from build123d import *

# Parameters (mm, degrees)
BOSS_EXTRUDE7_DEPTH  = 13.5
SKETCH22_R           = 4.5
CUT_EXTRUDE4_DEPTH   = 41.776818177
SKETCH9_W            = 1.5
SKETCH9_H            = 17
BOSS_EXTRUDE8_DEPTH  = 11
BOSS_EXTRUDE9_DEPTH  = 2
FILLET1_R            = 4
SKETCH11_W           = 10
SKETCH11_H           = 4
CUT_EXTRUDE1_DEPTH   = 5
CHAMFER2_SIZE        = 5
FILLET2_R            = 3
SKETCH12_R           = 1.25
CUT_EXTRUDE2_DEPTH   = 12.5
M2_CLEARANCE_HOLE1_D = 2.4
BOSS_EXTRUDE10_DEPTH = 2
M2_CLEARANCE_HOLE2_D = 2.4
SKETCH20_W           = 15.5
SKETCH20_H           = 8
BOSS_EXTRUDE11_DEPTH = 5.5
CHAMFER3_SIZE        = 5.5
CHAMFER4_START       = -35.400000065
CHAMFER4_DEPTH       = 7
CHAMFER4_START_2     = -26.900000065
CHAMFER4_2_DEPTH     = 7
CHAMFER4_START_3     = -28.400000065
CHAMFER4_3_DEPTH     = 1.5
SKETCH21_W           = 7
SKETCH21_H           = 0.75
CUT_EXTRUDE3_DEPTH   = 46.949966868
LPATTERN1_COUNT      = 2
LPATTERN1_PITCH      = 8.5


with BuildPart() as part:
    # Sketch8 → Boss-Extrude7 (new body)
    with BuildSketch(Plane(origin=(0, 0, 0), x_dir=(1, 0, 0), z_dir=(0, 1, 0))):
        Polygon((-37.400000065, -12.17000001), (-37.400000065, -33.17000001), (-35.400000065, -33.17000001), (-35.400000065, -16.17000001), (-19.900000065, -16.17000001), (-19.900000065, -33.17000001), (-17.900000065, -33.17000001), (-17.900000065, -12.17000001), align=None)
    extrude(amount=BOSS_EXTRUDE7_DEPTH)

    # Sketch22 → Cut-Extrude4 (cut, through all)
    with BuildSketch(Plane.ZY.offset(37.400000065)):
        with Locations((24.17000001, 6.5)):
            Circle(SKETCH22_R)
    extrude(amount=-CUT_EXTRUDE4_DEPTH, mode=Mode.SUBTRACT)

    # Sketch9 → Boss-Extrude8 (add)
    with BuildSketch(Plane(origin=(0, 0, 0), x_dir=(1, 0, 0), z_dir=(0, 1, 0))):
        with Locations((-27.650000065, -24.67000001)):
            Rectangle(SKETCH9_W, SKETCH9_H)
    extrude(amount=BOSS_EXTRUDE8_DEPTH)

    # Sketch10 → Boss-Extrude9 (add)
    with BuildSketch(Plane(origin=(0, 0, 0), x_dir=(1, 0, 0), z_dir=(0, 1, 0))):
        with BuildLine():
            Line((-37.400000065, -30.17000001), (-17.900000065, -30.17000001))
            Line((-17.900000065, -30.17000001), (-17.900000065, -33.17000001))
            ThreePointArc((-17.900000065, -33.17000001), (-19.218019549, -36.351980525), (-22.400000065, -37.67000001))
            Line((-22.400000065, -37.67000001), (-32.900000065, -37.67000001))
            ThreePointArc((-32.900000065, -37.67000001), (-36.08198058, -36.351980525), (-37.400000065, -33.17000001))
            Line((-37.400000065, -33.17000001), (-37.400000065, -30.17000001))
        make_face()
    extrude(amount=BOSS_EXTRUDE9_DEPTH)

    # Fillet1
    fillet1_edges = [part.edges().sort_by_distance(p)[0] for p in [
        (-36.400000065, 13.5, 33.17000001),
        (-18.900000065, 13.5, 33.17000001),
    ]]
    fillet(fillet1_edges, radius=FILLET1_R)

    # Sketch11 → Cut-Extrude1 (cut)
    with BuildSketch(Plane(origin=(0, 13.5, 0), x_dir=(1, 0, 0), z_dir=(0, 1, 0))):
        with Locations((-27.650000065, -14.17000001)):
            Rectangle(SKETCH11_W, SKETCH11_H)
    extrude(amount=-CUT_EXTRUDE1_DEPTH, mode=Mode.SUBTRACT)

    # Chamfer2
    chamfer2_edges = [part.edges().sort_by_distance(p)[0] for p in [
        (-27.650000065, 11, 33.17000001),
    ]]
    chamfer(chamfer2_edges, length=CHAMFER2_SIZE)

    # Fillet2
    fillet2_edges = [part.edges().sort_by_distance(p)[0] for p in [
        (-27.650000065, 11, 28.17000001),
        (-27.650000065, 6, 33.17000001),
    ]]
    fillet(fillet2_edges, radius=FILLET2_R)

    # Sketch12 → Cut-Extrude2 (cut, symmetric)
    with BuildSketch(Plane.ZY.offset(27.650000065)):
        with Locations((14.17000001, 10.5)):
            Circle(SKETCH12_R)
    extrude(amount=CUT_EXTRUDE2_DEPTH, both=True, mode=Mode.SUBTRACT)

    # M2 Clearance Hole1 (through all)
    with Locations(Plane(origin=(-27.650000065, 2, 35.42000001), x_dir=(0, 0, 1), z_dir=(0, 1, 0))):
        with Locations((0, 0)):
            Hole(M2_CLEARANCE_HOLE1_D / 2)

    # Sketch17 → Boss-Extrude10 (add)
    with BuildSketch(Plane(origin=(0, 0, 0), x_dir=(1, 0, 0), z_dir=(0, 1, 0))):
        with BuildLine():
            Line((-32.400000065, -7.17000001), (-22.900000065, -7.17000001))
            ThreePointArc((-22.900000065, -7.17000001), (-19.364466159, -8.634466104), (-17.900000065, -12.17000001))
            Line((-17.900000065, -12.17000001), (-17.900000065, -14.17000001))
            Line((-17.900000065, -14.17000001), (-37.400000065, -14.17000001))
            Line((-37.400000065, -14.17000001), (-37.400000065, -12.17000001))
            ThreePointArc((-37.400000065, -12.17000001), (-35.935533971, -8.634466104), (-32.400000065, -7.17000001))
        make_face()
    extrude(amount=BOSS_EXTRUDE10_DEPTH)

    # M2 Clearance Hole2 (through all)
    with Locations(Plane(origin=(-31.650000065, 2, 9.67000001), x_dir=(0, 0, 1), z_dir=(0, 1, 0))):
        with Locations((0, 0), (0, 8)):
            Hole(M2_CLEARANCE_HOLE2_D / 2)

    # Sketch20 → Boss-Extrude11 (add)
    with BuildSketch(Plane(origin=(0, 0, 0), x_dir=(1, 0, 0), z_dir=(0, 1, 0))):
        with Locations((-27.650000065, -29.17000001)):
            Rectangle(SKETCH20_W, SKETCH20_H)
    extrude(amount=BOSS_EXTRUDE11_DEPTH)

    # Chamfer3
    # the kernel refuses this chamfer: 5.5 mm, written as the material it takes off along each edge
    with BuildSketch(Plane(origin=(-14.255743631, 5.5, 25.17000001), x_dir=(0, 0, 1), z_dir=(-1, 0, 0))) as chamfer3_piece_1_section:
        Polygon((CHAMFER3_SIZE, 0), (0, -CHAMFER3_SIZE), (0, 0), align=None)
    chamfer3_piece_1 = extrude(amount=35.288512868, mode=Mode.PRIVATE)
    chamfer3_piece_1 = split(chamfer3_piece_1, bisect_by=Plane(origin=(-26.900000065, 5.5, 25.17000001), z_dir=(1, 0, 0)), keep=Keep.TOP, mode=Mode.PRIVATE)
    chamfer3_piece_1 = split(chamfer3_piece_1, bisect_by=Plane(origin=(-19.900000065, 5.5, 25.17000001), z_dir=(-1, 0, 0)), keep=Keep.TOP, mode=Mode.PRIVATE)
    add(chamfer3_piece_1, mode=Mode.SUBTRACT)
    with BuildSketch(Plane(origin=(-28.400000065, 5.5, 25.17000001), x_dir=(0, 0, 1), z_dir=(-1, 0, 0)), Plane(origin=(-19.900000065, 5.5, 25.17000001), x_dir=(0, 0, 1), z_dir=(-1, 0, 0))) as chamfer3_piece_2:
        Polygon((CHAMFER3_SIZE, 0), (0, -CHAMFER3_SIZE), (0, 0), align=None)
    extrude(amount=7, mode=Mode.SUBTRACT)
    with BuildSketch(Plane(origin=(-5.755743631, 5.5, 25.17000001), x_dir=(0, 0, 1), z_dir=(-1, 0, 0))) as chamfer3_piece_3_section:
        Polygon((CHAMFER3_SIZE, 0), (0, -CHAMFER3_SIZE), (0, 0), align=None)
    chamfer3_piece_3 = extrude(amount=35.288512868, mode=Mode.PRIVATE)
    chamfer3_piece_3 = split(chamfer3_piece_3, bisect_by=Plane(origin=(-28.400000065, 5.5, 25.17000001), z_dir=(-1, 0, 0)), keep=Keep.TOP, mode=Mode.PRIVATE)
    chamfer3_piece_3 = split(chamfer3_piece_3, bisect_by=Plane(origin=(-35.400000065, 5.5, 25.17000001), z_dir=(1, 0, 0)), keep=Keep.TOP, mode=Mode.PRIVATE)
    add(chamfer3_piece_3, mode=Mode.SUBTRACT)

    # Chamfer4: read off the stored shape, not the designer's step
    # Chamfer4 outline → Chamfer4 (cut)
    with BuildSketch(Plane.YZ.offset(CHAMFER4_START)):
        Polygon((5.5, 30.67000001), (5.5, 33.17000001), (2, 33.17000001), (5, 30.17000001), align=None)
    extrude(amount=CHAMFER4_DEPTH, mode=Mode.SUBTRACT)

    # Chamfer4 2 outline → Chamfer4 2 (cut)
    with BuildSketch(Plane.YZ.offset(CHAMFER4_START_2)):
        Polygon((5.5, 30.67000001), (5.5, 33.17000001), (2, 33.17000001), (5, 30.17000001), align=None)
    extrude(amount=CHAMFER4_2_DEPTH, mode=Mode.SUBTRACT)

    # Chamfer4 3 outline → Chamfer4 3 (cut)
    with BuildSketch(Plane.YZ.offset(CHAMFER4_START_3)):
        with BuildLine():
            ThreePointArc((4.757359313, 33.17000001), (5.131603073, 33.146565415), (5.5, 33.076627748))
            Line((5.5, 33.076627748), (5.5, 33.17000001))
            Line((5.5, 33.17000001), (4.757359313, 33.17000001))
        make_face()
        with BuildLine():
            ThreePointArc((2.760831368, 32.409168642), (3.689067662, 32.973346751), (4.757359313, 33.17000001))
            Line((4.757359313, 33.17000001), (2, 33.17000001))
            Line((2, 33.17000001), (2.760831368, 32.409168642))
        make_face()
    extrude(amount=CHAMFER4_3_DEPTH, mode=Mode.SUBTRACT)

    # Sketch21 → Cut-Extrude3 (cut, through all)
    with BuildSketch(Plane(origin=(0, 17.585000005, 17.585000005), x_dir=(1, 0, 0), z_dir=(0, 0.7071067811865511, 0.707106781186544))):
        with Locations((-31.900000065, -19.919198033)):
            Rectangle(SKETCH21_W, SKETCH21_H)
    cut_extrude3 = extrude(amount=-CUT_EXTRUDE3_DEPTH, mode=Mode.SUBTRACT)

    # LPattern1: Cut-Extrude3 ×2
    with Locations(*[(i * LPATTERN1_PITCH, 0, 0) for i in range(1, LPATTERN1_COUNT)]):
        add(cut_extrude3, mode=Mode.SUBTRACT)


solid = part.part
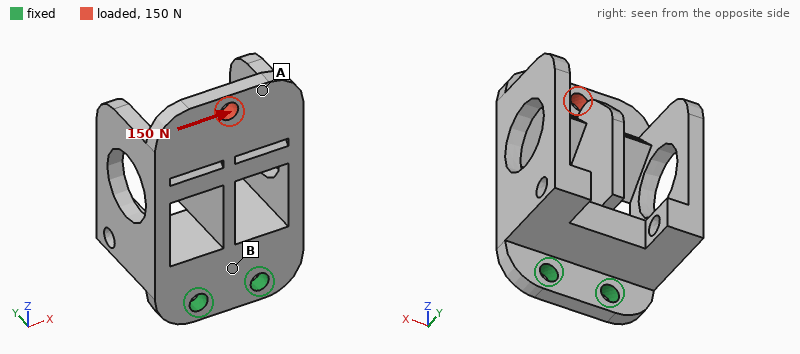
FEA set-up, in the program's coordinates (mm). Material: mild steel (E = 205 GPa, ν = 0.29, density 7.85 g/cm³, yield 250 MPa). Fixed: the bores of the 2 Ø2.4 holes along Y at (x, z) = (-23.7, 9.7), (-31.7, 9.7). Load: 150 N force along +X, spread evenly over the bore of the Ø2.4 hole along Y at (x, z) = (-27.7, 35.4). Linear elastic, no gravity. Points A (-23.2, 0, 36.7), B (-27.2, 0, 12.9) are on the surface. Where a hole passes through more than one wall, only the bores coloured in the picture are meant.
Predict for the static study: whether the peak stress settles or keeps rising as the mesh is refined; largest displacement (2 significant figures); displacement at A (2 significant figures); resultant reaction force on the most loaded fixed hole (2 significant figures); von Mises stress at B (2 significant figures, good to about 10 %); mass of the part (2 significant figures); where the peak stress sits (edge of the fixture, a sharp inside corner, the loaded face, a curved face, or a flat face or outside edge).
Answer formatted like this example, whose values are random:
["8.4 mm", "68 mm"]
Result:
["keeps rising", "26 µm", "25 µm", "370 N", "38 MPa", "18 g", "a sharp inside corner"]
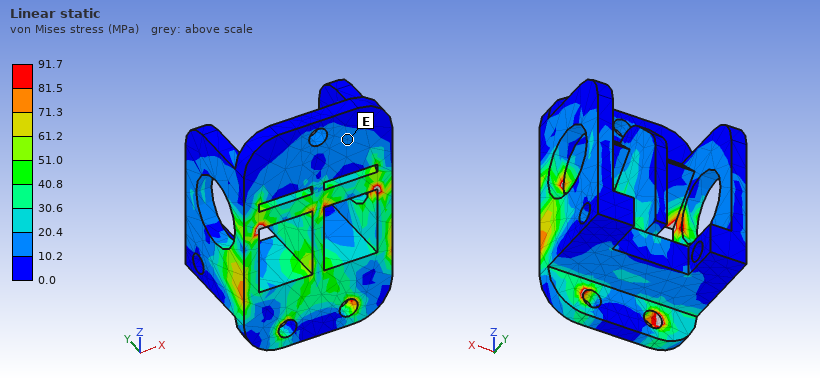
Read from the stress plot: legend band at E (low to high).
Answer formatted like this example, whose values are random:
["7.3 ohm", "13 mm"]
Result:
["10.2 to 20.4 MPa"]
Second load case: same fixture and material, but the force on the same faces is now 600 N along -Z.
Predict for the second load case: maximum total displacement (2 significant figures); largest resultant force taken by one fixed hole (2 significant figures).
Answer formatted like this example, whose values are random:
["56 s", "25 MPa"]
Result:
["13 µm", "300 N"]
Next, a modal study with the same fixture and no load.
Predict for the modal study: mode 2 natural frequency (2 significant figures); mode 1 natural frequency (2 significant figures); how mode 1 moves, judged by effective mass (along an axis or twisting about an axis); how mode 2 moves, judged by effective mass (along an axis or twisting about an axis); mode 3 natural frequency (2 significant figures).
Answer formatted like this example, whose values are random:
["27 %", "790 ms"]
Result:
["5400 Hz", "2400 Hz", "along Y", "along X", "6700 Hz"]
